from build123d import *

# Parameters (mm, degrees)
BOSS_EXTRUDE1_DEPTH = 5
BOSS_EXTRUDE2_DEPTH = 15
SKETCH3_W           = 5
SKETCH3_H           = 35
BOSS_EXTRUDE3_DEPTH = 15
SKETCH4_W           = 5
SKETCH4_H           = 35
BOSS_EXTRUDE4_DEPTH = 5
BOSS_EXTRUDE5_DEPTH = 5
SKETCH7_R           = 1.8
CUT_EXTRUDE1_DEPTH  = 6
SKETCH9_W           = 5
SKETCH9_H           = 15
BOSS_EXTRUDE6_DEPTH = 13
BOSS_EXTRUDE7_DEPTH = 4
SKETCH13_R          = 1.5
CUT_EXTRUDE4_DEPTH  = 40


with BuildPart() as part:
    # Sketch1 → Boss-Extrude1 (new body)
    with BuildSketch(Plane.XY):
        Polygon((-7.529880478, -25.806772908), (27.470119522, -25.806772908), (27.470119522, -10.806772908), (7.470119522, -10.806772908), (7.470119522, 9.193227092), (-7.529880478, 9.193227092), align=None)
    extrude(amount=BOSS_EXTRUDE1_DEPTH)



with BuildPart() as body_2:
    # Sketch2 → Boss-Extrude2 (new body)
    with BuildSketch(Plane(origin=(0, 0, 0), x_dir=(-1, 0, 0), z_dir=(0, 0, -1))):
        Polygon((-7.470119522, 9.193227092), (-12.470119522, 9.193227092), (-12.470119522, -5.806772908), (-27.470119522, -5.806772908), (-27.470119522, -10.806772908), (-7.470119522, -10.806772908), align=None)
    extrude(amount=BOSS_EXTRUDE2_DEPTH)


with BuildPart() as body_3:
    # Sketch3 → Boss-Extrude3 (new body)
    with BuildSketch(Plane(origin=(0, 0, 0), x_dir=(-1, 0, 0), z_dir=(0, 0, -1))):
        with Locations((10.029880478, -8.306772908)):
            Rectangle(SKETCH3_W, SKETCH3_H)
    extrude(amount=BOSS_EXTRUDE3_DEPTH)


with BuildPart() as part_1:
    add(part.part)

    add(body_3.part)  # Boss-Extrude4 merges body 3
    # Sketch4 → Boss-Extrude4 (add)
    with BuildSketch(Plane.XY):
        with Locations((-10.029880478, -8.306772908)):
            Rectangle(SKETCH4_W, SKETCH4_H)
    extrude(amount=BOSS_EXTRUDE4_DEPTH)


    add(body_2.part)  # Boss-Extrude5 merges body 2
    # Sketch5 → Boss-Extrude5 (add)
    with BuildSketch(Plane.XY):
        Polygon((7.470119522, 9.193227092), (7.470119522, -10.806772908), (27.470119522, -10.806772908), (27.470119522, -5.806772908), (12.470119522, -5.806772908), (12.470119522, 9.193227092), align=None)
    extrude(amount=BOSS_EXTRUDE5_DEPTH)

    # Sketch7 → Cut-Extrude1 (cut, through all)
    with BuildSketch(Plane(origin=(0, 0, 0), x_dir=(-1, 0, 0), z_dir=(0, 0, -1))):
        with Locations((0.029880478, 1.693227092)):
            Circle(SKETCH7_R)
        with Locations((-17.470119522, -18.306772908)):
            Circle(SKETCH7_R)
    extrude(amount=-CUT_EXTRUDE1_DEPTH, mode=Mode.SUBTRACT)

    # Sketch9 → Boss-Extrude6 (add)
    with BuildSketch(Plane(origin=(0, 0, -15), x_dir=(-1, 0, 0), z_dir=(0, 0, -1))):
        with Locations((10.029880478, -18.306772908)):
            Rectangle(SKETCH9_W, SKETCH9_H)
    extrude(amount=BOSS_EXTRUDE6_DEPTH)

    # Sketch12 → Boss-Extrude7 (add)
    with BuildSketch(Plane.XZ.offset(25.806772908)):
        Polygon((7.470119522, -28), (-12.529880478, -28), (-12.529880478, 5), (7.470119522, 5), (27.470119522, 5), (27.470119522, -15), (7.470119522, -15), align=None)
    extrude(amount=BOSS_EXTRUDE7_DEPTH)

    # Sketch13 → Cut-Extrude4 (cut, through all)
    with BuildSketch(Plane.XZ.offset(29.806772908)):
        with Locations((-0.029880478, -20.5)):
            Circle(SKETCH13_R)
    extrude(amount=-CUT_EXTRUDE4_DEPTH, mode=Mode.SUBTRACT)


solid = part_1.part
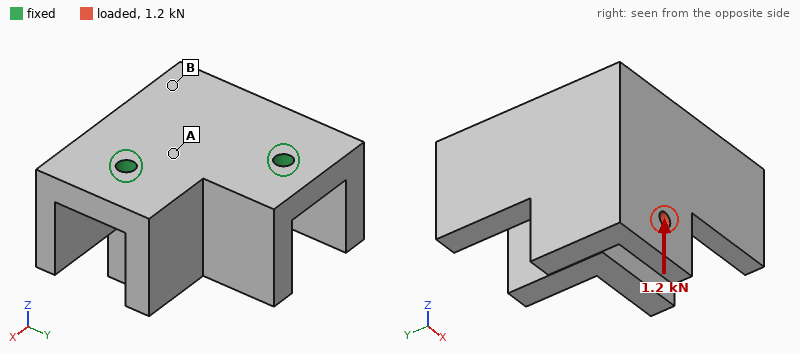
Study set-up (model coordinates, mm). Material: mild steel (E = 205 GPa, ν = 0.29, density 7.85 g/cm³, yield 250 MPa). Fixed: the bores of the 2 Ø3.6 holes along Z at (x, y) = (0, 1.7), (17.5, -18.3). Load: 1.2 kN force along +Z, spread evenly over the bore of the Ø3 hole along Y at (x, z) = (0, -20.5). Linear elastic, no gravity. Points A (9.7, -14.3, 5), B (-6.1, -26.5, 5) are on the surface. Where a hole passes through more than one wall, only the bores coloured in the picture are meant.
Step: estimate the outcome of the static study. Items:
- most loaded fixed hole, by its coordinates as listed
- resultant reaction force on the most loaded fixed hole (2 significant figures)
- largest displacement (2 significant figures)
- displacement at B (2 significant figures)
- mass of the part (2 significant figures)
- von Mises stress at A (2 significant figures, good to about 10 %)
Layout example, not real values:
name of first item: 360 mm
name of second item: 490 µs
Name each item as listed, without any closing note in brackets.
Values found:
most loaded fixed hole, by its coordinates as listed: (17.5, -18.3)
resultant reaction force on the most loaded fixed hole: 910 N
largest displacement: 82 µm
displacement at B: 40 µm
mass of the part: 130 g
von Mises stress at A: 56 MPa
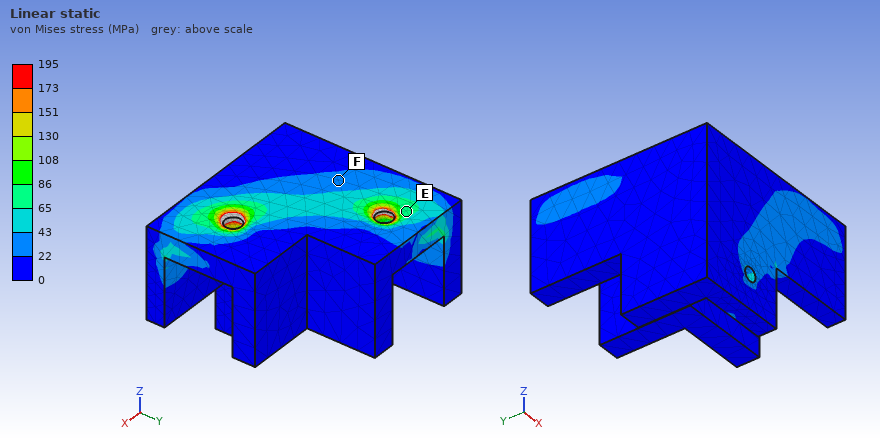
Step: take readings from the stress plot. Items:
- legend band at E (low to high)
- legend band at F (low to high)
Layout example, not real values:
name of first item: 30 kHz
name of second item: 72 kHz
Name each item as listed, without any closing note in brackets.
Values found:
legend band at E: 65 to 86 MPa
legend band at F: 22 to 43 MPa
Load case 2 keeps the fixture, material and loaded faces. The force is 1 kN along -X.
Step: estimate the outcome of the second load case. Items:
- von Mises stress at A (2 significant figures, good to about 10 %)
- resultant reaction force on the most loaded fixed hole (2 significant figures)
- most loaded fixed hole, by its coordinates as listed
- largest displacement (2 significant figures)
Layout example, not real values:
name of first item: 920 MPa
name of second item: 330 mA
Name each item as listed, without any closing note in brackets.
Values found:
von Mises stress at A: 46 MPa
resultant reaction force on the most loaded fixed hole: 1.2 kN
most loaded fixed hole, by its coordinates as listed: (17.5, -18.3)
largest displacement: 85 µm
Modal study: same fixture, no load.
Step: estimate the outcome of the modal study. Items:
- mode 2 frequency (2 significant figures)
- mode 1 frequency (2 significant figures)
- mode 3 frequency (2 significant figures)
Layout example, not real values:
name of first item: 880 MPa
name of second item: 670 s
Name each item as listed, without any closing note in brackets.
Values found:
mode 2 frequency: 6400 Hz
mode 1 frequency: 2900 Hz
mode 3 frequency: 9000 Hz
